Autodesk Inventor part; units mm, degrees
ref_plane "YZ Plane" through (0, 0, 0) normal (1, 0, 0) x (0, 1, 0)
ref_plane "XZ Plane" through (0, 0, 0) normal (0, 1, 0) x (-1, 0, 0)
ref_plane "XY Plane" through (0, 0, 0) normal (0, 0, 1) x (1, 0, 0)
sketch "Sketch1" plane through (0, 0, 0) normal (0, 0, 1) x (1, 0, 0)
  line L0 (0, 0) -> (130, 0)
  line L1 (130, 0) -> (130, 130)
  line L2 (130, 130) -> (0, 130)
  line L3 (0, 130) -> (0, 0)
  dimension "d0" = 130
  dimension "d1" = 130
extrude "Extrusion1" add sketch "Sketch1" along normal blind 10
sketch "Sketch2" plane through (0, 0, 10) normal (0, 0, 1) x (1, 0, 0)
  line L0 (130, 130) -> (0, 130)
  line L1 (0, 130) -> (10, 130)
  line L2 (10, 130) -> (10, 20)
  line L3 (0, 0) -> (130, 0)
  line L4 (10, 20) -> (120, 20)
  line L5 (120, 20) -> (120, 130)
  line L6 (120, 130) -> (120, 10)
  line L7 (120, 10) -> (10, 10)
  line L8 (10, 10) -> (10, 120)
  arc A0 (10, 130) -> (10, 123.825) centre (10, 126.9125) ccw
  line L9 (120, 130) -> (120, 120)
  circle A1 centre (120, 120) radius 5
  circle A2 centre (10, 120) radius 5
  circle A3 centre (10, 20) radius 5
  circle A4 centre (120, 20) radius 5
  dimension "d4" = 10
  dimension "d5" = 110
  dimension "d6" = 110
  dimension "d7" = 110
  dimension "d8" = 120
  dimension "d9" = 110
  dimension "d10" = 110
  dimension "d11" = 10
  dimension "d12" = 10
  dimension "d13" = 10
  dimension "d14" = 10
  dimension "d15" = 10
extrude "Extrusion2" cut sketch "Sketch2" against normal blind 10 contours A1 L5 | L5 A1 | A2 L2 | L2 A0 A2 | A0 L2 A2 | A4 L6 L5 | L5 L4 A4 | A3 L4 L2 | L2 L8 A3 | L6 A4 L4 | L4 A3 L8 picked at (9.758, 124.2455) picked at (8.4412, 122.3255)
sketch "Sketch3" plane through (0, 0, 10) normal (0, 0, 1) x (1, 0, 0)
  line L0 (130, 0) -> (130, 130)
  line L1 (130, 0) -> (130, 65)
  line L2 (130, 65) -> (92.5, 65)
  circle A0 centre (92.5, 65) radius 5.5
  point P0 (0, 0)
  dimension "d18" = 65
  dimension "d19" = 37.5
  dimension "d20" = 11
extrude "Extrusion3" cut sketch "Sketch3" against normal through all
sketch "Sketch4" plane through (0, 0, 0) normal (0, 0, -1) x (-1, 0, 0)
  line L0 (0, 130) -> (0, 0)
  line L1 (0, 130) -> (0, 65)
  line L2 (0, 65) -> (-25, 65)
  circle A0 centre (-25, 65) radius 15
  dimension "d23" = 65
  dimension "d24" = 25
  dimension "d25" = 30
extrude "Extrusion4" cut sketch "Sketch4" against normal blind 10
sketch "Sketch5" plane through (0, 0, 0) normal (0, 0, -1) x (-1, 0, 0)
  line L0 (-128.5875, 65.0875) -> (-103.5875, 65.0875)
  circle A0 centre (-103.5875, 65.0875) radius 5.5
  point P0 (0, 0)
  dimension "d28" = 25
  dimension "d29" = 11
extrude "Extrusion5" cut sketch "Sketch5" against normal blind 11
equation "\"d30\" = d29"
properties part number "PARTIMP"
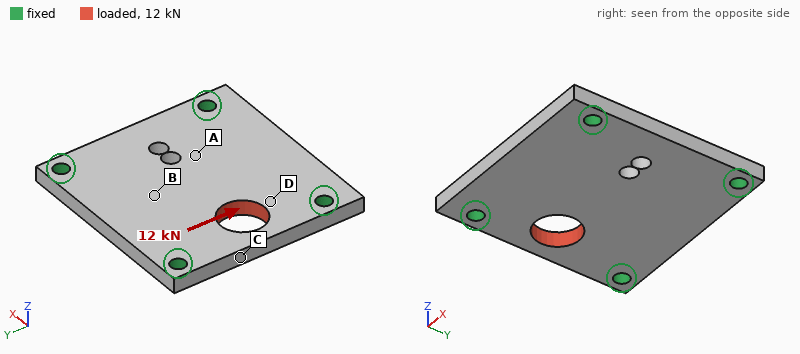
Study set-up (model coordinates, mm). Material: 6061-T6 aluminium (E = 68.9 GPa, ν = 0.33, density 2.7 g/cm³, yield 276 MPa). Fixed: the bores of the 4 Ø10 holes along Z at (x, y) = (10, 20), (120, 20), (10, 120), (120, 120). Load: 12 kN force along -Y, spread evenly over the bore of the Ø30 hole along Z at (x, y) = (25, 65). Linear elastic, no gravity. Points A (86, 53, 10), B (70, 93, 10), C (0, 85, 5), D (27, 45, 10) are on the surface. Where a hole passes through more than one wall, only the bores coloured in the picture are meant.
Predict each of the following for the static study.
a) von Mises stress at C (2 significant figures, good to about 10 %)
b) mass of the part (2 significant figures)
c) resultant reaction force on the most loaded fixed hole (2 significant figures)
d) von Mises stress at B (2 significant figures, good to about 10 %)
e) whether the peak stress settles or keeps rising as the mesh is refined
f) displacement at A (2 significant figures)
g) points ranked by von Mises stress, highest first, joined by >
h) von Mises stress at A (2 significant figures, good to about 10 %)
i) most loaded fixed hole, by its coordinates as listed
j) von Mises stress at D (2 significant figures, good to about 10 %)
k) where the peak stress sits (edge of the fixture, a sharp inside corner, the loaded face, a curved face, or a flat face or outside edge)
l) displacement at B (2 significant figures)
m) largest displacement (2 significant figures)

10 MPa
420 g
5.2 kN
4.7 MPa
keeps rising
4.2 µm
D > C > B > A
2.9 MPa
(10, 20)
15 MPa
edge of the fixture
6.1 µm
12 µm
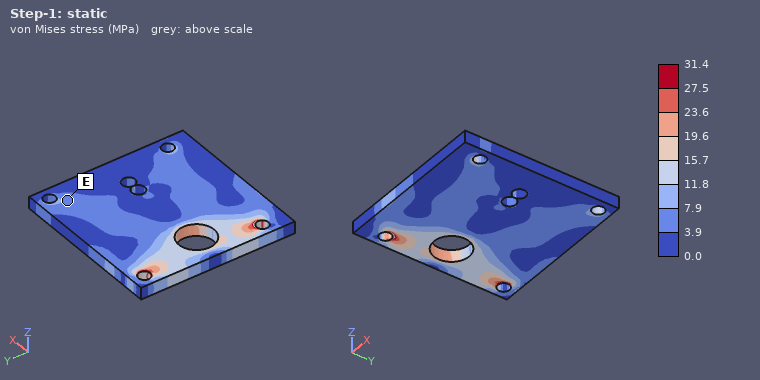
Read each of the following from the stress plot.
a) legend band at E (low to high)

3.9 to 7.9 MPa
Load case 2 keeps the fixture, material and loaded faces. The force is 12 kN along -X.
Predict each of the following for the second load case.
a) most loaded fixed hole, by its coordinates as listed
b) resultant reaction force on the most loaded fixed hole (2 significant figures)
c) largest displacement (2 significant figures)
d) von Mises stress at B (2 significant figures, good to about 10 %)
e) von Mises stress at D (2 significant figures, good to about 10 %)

(10, 20)
4.1 kN
30 µm
9.2 MPa
25 MPa
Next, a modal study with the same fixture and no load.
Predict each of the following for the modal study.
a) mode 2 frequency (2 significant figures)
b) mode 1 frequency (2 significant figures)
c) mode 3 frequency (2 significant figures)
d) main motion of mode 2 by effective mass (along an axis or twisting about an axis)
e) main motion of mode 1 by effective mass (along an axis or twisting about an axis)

4600 Hz
3100 Hz
5400 Hz
twisting about X
along Z
